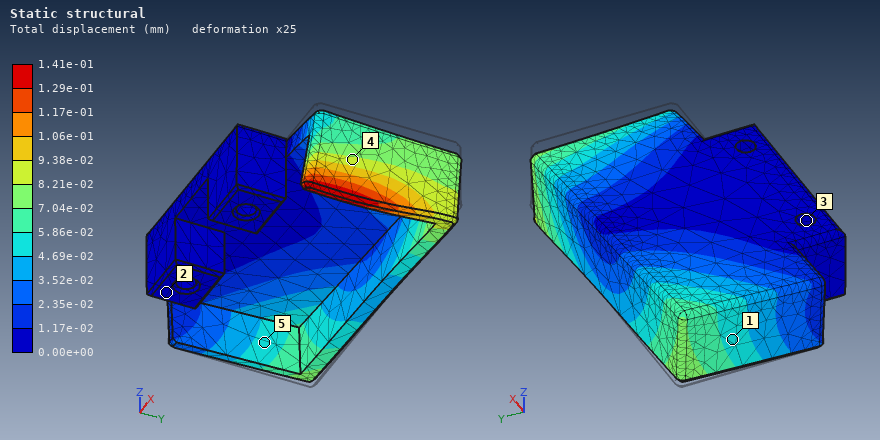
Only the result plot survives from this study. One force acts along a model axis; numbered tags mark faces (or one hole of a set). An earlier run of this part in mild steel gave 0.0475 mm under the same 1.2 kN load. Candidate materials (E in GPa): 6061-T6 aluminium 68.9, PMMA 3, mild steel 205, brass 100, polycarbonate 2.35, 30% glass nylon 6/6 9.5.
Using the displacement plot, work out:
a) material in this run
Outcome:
6061-T6 aluminium
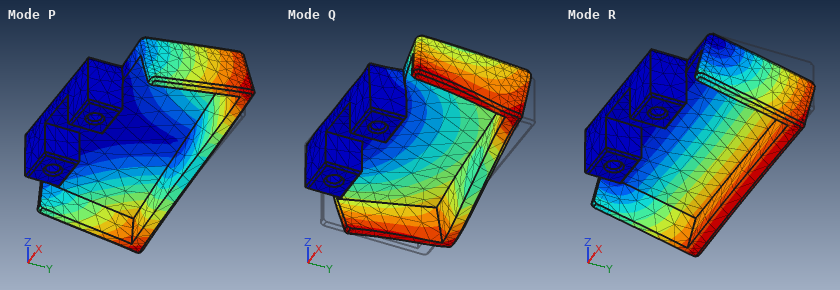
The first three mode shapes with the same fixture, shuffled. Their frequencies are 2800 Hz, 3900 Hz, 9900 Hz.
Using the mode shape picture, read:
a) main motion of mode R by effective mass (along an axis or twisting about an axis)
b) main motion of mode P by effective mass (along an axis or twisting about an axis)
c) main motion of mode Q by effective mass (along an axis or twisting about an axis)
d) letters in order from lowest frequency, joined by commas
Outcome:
along Z
twisting about Y
along X
R, P, Q
